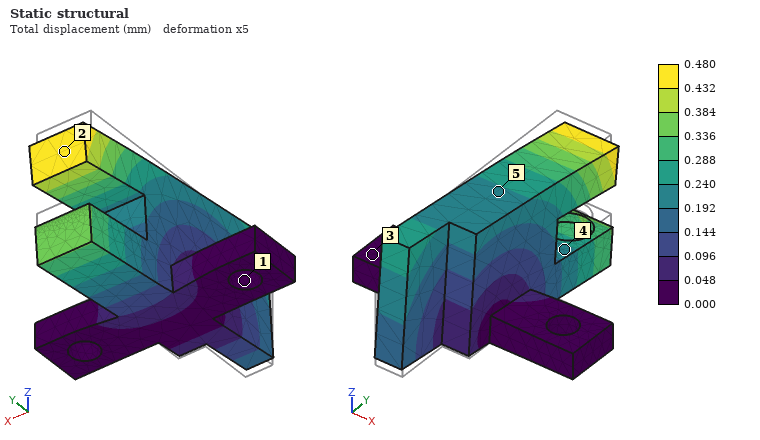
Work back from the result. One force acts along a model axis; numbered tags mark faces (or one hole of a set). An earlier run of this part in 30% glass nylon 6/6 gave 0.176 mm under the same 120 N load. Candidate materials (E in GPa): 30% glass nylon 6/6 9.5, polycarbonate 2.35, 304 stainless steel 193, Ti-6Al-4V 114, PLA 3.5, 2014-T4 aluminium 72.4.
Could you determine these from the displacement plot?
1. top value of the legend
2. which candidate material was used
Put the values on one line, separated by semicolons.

0.480 mm; PLA
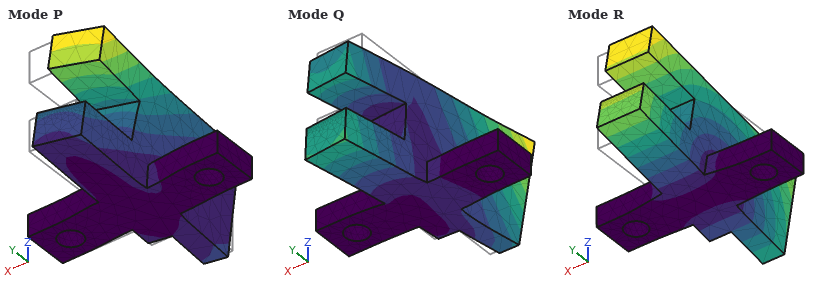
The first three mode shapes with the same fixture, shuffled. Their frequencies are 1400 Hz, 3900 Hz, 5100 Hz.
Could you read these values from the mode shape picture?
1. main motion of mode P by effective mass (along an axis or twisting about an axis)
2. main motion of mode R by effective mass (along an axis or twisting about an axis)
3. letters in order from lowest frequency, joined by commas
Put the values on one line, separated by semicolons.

along X; along Y; R, P, Q
